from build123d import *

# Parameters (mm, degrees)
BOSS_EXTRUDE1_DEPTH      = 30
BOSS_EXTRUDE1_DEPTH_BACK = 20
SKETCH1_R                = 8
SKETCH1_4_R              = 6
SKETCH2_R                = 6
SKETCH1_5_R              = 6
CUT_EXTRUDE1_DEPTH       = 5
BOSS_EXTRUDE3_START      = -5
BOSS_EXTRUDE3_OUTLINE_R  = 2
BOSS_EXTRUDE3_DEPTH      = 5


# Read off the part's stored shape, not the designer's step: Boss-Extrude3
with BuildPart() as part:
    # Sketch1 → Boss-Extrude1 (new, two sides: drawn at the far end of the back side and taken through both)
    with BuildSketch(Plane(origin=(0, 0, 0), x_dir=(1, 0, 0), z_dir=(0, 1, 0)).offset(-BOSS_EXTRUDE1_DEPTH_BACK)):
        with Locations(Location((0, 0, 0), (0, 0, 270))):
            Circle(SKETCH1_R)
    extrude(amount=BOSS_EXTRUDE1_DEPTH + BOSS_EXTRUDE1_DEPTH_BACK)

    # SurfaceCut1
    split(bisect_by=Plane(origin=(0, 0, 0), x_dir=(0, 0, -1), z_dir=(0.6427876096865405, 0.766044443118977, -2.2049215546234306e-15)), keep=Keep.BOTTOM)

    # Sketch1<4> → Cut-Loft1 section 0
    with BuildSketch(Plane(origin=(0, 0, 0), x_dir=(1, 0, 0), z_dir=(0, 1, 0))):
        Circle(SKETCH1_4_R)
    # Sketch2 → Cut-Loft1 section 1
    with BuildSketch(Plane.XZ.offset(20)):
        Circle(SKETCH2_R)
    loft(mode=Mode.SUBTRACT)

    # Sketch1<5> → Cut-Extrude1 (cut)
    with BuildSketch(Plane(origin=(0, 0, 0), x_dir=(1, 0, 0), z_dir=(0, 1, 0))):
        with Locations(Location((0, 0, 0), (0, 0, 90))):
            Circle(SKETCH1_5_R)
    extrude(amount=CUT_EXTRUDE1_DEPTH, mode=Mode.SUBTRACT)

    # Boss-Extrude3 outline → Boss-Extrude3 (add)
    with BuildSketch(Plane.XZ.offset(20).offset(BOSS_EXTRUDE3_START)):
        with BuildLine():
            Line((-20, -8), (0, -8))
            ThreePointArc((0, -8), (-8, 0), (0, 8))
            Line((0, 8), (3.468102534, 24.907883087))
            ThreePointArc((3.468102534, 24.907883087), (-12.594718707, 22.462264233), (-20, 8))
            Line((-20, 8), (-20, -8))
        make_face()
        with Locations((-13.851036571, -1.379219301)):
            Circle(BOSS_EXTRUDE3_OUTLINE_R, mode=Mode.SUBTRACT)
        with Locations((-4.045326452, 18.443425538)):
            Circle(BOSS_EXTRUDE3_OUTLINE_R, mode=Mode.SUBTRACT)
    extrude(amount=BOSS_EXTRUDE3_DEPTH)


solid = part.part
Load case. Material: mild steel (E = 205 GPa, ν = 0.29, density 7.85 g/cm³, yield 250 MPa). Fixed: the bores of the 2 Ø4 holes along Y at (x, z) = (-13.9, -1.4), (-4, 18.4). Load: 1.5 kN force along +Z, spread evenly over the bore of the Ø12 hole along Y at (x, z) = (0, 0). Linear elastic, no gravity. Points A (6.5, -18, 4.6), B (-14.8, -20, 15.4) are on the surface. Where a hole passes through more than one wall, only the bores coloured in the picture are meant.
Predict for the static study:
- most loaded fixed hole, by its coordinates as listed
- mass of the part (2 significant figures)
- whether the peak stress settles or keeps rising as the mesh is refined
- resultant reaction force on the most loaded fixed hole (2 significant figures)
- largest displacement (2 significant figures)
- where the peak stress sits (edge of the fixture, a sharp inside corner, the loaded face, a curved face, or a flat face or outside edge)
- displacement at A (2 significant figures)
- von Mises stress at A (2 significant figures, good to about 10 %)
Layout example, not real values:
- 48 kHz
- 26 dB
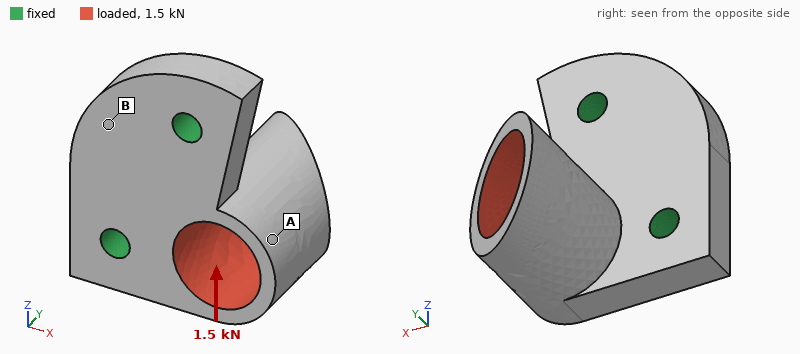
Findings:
- (-4, 18.4)
- 34 g
- keeps rising
- 1.1 kN
- 38 µm
- edge of the fixture
- 14 µm
- 55 MPa
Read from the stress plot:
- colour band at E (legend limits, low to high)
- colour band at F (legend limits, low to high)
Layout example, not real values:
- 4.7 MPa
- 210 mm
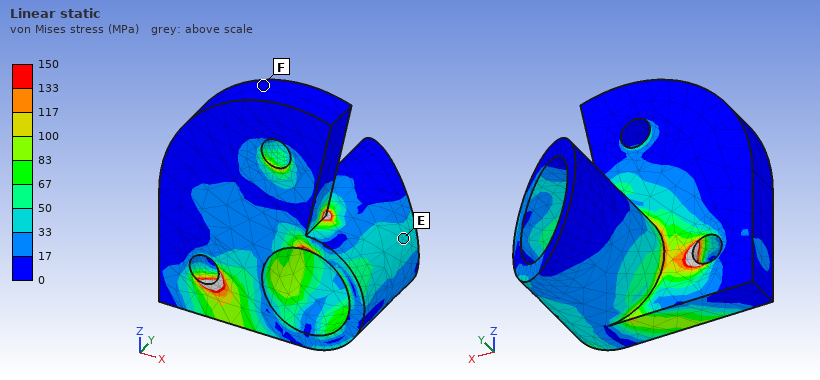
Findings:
- 33 to 50 MPa
- 0 to 17 MPa
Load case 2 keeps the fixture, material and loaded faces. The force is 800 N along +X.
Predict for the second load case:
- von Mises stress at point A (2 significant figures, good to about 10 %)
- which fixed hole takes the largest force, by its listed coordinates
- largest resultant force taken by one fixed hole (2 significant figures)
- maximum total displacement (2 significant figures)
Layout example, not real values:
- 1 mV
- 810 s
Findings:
- 13 MPa
- (-13.9, -1.4)
- 710 N
- 38 µm
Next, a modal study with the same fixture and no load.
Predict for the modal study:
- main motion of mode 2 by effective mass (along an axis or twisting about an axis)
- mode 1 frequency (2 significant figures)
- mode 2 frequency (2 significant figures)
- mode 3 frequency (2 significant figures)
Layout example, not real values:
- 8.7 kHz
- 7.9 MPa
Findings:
- along Z
- 6400 Hz
- 11 kHz
- 17 kHz
